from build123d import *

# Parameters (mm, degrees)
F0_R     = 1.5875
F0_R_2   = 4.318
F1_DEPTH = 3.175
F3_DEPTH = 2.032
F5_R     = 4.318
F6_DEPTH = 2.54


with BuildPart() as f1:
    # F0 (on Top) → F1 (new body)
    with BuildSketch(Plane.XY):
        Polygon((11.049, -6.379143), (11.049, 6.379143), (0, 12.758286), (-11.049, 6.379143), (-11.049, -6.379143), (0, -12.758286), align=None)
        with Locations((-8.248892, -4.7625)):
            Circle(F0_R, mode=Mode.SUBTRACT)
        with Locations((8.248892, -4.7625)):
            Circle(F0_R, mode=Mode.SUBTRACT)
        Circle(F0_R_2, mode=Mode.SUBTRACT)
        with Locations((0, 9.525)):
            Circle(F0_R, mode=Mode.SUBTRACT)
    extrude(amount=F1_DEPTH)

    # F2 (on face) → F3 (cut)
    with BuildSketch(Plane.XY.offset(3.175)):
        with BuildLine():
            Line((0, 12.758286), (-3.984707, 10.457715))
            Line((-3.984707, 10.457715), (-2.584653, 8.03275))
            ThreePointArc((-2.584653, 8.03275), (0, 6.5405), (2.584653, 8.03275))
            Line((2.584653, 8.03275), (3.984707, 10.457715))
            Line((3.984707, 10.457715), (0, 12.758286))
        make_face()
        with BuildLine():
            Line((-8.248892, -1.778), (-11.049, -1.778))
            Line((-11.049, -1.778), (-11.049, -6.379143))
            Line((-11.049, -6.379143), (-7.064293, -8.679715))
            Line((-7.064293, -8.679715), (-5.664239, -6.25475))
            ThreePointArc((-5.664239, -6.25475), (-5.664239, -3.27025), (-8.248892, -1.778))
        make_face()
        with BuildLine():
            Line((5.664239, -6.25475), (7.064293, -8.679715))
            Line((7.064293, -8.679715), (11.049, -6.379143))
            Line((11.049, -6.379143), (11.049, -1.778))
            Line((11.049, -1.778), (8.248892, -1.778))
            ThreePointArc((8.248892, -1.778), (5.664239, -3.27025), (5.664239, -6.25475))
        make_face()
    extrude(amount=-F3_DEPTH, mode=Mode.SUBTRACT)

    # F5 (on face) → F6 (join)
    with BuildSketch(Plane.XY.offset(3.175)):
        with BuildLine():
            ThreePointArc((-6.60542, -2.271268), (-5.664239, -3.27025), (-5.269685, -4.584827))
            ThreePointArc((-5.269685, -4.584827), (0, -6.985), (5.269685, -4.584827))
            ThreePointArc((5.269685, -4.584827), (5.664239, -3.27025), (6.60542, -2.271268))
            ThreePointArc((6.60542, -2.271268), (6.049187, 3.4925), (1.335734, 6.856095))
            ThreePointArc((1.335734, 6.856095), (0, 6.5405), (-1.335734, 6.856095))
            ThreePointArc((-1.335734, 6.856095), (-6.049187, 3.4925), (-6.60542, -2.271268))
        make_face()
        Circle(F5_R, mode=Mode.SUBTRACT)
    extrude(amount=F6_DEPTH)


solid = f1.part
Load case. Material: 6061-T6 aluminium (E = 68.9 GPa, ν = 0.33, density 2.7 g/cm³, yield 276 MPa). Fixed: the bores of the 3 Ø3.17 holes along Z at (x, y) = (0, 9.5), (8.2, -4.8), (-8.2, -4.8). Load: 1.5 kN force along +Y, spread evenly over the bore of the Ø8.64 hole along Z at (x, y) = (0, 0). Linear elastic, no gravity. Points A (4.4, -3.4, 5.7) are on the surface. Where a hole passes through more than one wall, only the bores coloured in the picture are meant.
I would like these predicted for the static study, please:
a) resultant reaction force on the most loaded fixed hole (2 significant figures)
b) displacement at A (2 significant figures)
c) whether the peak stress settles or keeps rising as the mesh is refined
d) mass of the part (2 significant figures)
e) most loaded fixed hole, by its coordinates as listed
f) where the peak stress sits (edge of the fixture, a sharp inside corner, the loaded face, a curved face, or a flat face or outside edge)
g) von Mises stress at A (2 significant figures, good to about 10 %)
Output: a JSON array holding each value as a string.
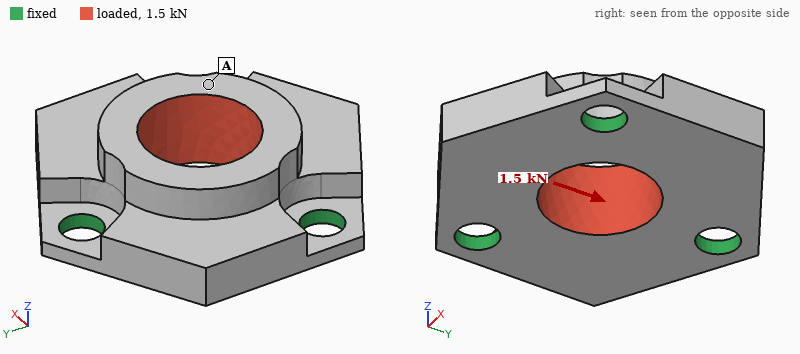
["600 N", "9.0 µm", "keeps rising", "3.2 g", "(0, 9.5)", "edge of the fixture", "19 MPa"]
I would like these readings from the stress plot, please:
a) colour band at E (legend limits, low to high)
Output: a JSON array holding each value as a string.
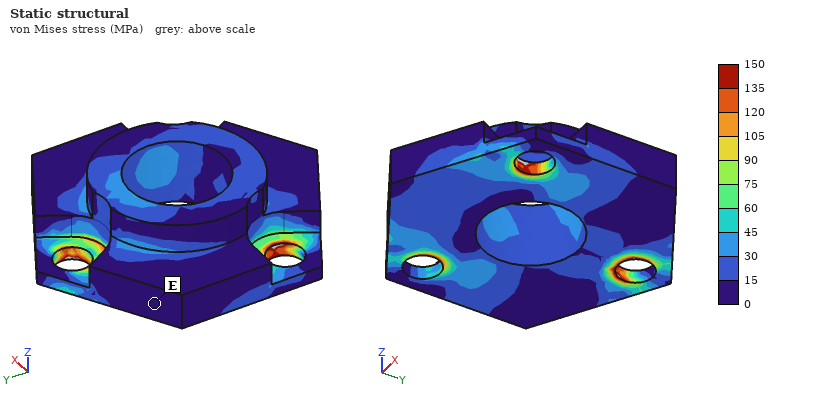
["0 to 15 MPa"]
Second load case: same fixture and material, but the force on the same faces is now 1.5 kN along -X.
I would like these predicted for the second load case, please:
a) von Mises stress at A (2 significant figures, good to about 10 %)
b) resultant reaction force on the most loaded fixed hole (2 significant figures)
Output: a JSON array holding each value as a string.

["27 MPa", "570 N"]
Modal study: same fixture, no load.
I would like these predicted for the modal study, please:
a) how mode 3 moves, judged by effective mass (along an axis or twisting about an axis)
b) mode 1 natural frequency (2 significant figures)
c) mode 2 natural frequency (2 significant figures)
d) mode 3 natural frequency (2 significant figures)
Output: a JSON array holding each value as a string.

["along Z", "27 kHz", "27 kHz", "33 kHz"]
